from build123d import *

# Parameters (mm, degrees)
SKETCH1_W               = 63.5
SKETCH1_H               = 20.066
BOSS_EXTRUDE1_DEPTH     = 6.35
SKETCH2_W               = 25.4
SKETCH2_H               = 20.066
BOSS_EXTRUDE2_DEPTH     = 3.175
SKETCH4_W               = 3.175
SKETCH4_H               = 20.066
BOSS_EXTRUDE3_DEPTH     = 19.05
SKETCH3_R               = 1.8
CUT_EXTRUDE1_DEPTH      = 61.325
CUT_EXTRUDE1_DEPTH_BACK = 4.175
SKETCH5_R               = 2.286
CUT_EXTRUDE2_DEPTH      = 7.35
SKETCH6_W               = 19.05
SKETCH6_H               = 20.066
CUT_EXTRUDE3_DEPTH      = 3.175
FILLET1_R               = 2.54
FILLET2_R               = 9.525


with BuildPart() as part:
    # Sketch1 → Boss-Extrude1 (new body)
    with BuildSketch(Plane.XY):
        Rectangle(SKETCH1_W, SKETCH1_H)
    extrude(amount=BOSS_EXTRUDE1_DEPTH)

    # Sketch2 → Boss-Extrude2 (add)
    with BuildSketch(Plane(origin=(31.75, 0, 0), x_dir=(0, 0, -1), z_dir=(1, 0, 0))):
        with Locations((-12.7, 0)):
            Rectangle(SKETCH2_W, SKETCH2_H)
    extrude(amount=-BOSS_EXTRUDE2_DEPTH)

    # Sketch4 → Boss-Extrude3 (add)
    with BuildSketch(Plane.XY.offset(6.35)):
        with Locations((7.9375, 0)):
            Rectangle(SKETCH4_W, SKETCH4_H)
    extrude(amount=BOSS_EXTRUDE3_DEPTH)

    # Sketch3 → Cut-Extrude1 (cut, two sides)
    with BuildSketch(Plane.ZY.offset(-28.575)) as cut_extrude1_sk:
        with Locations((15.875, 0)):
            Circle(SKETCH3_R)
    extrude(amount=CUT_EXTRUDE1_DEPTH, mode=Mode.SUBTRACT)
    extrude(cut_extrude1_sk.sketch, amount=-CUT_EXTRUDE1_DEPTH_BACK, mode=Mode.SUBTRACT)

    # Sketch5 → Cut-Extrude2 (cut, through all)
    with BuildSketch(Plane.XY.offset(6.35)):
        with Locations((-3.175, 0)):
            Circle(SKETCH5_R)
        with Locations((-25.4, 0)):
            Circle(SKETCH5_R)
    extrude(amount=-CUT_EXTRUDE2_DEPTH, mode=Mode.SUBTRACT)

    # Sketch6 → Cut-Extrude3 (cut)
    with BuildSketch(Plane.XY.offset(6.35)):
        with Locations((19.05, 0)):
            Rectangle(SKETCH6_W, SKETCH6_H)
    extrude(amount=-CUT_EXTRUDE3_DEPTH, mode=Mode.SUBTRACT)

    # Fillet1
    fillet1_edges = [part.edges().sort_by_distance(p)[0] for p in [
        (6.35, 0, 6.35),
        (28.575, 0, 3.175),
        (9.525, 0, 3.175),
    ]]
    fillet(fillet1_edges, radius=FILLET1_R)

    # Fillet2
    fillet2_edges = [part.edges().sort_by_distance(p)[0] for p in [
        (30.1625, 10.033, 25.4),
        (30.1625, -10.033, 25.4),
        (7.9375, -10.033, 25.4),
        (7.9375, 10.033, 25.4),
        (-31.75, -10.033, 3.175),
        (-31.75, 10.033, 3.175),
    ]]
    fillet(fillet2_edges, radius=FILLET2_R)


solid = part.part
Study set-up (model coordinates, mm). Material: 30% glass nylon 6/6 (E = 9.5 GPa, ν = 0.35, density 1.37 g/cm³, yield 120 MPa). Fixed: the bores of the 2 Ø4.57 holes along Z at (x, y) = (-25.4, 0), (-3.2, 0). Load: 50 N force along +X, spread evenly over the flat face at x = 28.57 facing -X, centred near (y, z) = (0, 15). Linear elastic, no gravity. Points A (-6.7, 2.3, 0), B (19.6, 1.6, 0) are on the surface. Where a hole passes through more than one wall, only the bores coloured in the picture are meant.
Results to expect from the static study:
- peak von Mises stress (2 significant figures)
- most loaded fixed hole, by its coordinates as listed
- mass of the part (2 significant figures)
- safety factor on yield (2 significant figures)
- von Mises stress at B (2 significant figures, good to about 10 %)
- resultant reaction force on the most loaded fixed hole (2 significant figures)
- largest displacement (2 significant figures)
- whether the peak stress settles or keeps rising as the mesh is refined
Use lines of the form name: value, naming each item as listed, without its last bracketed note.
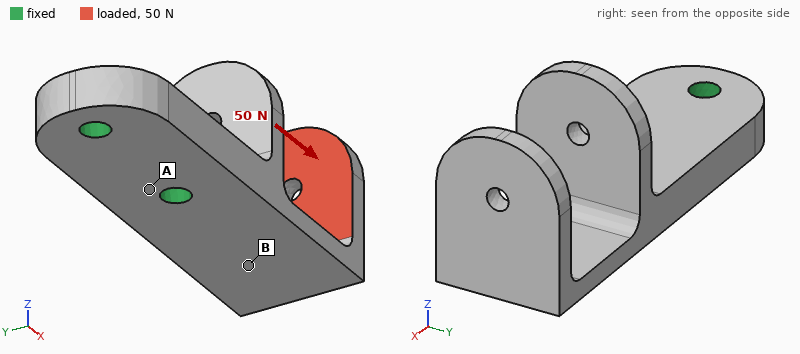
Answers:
peak von Mises stress: 22 MPa
most loaded fixed hole, by its coordinates as listed: (-3.2, 0)
mass of the part: 12 g
safety factor on yield: 5.4
von Mises stress at B: 16 MPa
resultant reaction force on the most loaded fixed hole: 44 N
largest displacement: 0.79 mm
whether the peak stress settles or keeps rising as the mesh is refined: settles
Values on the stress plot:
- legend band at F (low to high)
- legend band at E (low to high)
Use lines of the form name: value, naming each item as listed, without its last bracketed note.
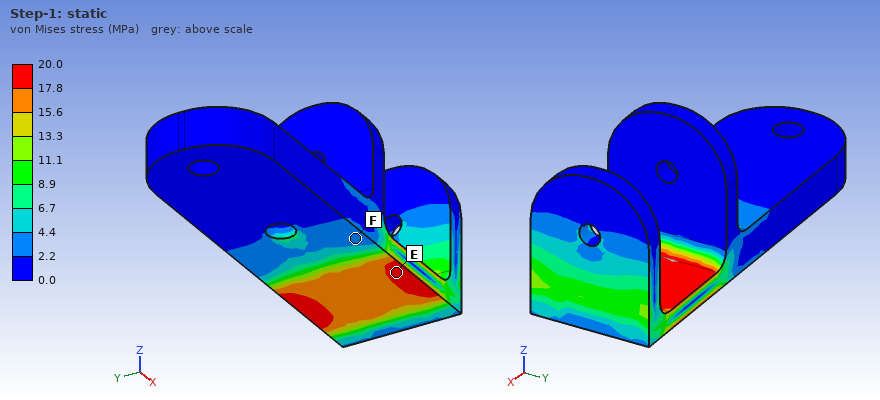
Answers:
legend band at F: 2.2 to 4.4 MPa
legend band at E: 17.8 to 20.0 MPa
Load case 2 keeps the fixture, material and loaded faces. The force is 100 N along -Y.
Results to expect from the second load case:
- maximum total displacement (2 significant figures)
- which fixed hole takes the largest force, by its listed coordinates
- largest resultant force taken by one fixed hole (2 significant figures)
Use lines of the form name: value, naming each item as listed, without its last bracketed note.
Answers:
maximum total displacement: 0.79 mm
which fixed hole takes the largest force, by its listed coordinates: (-3.2, 0)
largest resultant force taken by one fixed hole: 190 N
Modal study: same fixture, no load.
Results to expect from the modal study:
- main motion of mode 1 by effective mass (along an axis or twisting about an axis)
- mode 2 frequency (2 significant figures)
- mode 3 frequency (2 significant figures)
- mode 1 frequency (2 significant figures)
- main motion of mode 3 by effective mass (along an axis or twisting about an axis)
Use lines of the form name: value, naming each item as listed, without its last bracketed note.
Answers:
main motion of mode 1 by effective mass: along Z
mode 2 frequency: 1600 Hz
mode 3 frequency: 2500 Hz
mode 1 frequency: 940 Hz
main motion of mode 3 by effective mass: along Z
